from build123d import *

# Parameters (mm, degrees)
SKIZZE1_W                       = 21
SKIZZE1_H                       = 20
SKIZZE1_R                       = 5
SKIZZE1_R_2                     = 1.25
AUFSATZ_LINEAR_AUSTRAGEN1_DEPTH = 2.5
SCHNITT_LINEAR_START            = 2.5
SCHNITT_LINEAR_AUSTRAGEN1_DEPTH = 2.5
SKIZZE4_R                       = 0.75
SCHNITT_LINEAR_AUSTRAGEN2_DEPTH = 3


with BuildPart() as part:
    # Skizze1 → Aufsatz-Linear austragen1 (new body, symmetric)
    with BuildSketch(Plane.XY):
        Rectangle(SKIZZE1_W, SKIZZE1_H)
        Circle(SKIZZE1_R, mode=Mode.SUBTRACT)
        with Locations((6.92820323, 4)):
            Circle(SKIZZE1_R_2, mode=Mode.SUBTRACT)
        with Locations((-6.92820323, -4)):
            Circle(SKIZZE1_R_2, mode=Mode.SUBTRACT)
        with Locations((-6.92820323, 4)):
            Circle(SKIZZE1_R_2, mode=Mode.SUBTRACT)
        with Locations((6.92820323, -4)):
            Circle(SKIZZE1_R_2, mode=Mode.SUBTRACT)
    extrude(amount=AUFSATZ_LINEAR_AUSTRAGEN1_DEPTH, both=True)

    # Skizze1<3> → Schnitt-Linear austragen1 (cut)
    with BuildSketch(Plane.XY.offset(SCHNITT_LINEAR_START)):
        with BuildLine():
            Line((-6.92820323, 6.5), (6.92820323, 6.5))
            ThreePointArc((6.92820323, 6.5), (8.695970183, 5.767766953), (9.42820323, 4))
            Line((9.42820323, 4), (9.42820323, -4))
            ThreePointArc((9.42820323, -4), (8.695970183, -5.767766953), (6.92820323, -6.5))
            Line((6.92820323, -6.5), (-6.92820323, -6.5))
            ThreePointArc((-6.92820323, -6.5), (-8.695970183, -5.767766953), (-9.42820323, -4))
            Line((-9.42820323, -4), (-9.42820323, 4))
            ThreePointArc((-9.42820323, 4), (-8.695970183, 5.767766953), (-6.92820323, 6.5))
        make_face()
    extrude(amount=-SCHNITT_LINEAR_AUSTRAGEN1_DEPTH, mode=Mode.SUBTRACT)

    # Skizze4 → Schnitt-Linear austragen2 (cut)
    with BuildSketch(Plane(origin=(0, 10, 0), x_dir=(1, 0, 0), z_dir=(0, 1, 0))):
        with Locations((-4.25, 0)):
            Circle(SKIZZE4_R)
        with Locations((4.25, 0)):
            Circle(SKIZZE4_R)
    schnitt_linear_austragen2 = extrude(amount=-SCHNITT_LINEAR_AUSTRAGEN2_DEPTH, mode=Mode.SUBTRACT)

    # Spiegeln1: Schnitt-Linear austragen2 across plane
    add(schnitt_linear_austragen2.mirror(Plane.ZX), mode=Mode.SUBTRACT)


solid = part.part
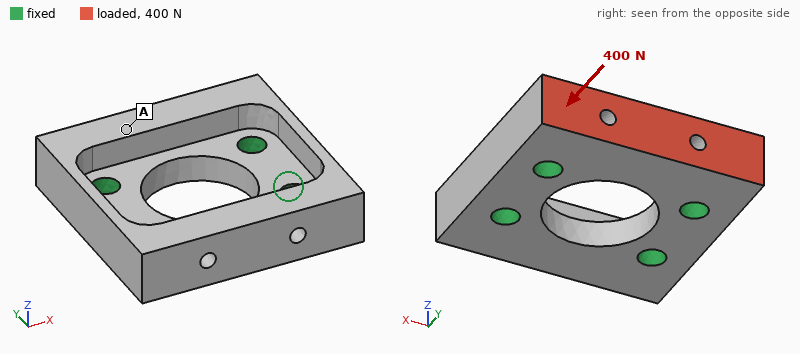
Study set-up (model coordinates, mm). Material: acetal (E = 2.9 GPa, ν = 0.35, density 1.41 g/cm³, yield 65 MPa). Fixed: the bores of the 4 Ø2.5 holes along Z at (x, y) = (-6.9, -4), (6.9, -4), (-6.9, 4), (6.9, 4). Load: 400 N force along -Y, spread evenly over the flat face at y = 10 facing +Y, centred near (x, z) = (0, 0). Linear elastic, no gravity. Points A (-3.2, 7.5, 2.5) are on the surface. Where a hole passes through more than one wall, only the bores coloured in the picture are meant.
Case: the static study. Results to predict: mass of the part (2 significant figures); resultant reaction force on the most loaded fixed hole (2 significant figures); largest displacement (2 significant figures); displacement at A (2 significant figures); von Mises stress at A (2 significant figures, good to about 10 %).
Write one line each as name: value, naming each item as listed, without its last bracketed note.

mass of the part: 1.7 g
resultant reaction force on the most loaded fixed hole: 190 N
largest displacement: 0.13 mm
displacement at A: 0.097 mm
von Mises stress at A: 4.7 MPa
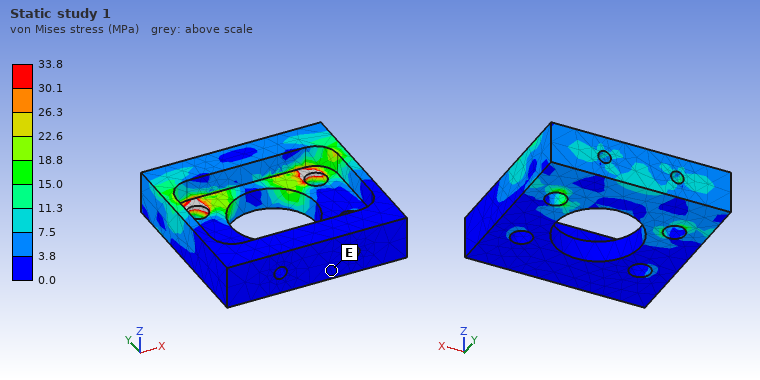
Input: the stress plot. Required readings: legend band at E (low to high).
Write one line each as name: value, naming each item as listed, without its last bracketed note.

legend band at E: 0.0 to 3.8 MPa
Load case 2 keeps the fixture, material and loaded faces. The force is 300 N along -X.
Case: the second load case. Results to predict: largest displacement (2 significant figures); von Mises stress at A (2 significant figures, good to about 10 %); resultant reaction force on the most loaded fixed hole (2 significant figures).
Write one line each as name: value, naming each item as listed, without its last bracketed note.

largest displacement: 59 µm
von Mises stress at A: 5.0 MPa
resultant reaction force on the most loaded fixed hole: 180 N
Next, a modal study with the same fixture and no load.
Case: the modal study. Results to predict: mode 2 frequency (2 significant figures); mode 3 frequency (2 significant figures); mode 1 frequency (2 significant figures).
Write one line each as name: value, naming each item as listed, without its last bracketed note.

mode 2 frequency: 10 kHz
mode 3 frequency: 15 kHz
mode 1 frequency: 10 kHz
